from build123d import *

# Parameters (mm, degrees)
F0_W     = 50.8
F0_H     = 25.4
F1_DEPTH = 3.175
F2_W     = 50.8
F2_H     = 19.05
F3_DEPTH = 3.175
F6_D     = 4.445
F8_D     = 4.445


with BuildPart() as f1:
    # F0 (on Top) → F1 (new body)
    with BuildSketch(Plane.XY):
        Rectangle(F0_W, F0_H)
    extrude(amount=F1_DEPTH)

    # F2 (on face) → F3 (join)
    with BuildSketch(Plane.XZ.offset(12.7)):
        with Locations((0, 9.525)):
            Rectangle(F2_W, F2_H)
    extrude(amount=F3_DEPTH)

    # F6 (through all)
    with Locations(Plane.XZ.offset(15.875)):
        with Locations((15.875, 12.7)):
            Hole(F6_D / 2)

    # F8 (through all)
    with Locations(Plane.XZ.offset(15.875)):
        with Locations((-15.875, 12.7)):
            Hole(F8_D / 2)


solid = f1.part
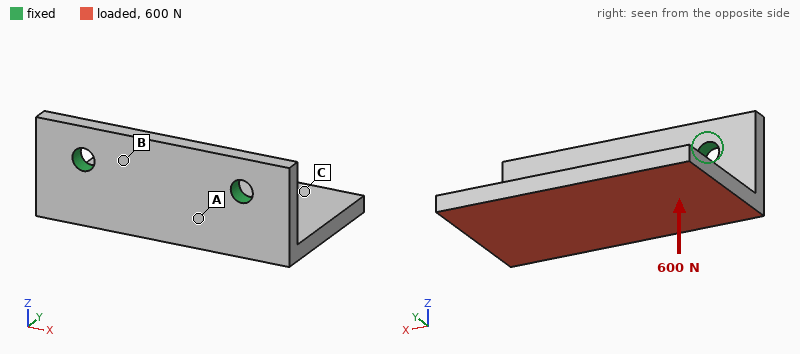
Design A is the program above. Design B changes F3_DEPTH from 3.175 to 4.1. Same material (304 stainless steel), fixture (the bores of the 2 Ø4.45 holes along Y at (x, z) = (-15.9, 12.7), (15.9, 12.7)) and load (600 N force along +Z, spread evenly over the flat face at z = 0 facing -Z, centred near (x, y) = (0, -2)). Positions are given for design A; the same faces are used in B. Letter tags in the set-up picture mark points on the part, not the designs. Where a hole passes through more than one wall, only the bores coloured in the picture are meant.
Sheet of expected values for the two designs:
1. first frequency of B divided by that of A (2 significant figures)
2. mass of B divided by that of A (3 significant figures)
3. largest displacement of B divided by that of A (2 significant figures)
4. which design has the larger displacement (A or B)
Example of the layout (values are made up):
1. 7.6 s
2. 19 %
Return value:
1. 1.2
2. 1.12
3. 0.67
4. A
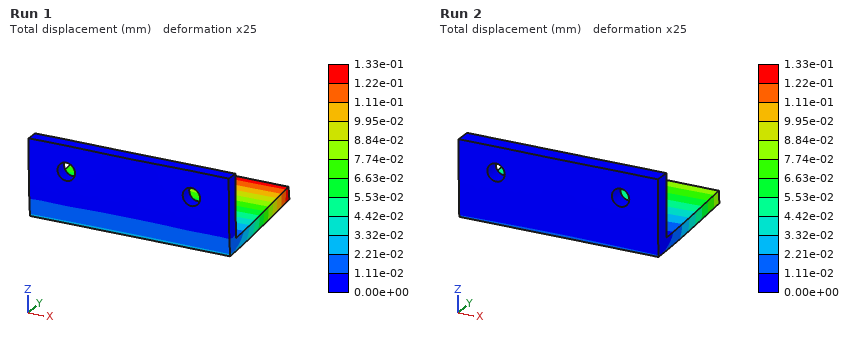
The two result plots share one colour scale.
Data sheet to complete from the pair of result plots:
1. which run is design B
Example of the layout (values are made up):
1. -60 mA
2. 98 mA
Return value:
1. Run 2
